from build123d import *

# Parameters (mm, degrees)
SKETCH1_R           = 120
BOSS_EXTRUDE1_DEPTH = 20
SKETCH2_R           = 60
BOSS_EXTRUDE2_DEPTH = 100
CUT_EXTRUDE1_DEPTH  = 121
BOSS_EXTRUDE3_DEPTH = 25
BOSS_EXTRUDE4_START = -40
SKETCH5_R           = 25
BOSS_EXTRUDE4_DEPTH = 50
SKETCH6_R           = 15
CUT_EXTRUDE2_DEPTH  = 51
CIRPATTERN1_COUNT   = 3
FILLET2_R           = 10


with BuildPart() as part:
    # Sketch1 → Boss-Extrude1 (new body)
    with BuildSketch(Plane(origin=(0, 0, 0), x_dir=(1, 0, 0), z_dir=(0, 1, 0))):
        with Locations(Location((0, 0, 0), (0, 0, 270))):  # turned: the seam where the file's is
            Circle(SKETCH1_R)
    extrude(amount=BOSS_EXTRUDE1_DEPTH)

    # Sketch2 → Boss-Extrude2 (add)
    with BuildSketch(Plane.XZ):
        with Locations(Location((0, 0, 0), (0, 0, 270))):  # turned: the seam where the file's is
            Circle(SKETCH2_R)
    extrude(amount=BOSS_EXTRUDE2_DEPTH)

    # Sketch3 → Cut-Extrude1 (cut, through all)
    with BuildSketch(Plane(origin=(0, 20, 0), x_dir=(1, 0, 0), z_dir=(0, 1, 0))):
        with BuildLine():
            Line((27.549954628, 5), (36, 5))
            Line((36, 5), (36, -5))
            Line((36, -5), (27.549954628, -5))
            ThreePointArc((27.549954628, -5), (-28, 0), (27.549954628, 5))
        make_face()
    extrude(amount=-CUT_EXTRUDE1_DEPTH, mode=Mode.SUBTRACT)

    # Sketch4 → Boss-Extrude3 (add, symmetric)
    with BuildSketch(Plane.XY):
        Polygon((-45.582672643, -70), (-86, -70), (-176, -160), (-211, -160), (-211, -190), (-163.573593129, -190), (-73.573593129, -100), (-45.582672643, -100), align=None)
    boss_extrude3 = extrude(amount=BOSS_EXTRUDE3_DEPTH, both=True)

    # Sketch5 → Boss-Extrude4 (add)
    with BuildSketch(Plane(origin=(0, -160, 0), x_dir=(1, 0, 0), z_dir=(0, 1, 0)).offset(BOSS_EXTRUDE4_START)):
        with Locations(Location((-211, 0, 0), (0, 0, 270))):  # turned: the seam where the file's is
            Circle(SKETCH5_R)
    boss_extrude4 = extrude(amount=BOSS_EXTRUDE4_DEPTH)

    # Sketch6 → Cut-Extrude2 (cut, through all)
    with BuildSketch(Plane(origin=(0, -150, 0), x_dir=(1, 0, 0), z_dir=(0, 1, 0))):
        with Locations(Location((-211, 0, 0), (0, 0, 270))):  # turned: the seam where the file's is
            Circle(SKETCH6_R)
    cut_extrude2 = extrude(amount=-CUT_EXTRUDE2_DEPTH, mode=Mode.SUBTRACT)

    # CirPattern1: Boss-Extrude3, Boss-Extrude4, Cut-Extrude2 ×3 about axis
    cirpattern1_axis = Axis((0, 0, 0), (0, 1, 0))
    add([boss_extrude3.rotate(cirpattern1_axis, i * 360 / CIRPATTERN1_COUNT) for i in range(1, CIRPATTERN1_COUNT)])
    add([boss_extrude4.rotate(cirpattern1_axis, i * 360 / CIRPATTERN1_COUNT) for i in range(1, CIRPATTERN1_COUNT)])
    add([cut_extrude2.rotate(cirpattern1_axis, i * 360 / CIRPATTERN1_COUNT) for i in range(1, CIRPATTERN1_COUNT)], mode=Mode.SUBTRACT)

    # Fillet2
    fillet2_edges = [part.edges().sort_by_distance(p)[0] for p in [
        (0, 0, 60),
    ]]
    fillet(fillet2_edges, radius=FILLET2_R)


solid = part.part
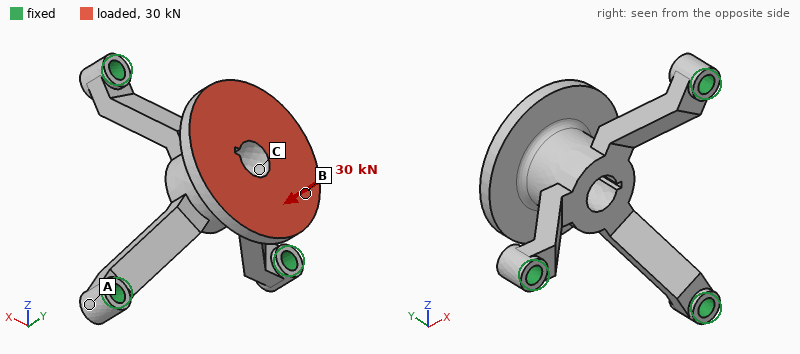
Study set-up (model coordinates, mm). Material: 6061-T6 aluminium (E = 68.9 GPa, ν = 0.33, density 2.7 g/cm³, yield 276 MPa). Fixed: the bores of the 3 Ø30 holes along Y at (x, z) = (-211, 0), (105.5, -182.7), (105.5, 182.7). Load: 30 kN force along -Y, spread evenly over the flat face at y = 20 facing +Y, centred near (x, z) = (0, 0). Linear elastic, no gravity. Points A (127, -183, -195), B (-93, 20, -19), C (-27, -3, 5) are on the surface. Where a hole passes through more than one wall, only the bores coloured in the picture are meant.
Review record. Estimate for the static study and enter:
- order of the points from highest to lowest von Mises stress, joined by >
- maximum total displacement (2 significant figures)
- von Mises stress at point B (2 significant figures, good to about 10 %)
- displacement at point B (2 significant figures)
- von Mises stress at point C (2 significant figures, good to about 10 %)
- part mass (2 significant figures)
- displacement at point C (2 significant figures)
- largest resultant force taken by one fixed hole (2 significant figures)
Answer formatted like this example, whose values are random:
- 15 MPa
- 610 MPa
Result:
- B > C > A
- 0.11 mm
- 7.1 MPa
- 0.090 mm
- 4.2 MPa
- 7.3 kg
- 0.060 mm
- 15 kN
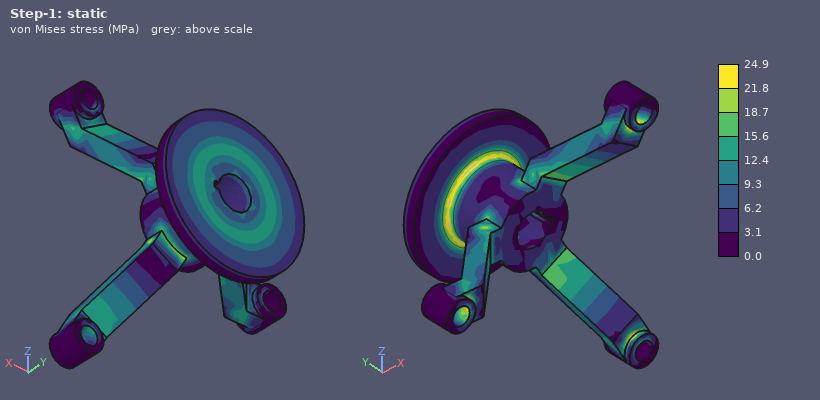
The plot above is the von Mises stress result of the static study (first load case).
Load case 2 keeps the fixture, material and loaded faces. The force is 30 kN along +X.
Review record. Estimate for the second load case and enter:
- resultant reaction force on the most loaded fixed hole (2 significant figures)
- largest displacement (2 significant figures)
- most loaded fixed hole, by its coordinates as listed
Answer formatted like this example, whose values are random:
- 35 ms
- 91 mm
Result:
- 32 kN
- 0.37 mm
- (-211, 0)
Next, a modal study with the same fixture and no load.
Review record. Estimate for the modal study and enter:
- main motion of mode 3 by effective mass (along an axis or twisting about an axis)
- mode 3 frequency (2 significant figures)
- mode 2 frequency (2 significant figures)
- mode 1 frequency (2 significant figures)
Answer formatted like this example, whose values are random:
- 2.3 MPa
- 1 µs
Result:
- twisting about Y
- 1100 Hz
- 950 Hz
- 950 Hz
